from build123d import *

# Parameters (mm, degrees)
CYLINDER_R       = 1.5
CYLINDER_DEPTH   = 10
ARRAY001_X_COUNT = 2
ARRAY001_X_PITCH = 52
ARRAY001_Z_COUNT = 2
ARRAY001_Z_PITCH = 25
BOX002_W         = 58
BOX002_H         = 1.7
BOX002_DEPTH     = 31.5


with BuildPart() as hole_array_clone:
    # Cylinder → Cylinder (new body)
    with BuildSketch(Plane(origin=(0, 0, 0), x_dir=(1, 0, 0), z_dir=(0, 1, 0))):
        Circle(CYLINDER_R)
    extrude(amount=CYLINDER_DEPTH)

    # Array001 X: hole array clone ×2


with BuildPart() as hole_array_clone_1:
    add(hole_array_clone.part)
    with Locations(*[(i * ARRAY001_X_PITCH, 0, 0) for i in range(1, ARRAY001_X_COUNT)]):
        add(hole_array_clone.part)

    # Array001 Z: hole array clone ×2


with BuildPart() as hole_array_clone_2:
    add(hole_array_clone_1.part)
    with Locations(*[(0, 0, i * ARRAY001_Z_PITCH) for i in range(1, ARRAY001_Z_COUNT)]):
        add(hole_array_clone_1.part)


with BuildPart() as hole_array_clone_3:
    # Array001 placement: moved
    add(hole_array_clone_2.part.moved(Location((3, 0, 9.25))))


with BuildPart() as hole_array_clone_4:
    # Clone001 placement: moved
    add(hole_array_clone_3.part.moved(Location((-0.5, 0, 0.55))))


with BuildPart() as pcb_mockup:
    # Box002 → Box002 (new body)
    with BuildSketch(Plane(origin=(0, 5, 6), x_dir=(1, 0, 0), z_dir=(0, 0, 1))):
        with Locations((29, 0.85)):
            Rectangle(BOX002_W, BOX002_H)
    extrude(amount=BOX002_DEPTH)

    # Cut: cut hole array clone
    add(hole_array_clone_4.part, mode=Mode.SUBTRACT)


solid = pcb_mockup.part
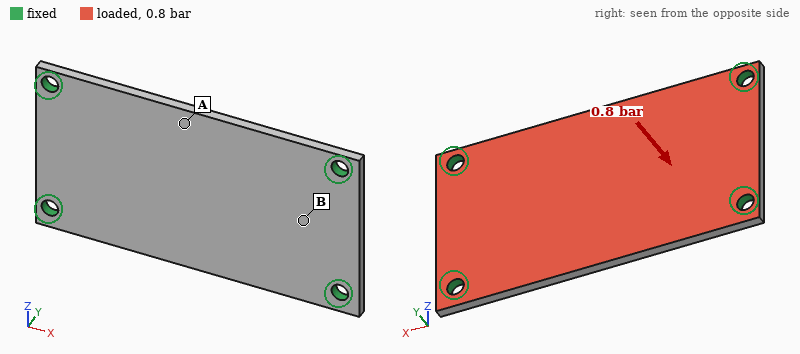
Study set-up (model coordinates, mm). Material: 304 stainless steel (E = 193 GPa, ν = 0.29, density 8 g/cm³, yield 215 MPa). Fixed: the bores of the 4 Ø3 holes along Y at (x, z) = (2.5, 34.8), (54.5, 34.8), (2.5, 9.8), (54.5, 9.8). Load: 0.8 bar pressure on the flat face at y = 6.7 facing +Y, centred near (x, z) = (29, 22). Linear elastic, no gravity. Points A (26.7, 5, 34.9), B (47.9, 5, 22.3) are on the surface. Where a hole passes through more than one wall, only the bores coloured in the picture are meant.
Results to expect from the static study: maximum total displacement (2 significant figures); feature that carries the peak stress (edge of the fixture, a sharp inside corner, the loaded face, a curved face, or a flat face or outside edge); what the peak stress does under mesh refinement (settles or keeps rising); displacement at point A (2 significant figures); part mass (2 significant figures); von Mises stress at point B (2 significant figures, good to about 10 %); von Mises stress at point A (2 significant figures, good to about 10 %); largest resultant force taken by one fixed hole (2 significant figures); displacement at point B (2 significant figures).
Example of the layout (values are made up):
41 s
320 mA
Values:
22 µm
edge of the fixture
keeps rising
21 µm
24 g
10 MPa
20 MPa
38 N
6.6 µm
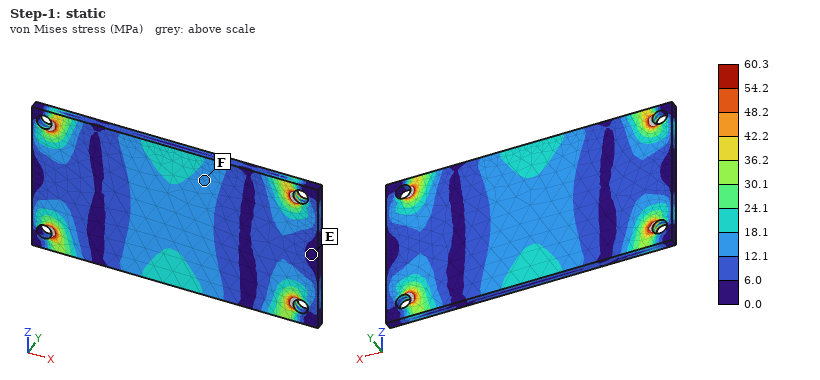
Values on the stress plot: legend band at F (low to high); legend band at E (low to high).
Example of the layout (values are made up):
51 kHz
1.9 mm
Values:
12.1 to 18.1 MPa
0.0 to 6.0 MPa
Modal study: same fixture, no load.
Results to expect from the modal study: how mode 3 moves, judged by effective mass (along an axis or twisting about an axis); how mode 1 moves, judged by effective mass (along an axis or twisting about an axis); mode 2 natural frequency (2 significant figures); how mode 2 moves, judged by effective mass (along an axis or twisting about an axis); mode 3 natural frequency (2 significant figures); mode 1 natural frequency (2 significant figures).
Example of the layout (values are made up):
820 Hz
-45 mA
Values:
twisting about Z
along Y
4900 Hz
twisting about X
8100 Hz
3000 Hz
